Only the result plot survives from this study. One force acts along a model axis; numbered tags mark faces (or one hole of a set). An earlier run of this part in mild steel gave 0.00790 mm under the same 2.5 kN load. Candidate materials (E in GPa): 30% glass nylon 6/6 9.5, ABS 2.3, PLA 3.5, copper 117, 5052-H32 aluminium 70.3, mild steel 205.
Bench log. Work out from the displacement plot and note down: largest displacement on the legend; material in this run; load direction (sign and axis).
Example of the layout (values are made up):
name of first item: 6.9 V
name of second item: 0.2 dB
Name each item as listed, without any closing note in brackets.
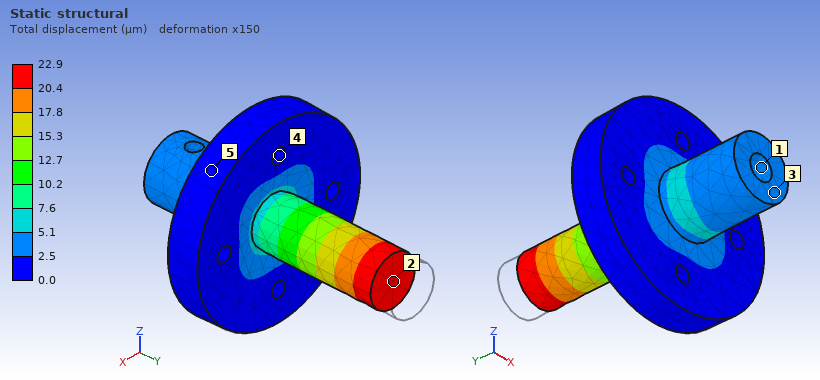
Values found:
largest displacement on the legend: 22.9 µm
material in this run: 5052-H32 aluminium
load direction: -Y
